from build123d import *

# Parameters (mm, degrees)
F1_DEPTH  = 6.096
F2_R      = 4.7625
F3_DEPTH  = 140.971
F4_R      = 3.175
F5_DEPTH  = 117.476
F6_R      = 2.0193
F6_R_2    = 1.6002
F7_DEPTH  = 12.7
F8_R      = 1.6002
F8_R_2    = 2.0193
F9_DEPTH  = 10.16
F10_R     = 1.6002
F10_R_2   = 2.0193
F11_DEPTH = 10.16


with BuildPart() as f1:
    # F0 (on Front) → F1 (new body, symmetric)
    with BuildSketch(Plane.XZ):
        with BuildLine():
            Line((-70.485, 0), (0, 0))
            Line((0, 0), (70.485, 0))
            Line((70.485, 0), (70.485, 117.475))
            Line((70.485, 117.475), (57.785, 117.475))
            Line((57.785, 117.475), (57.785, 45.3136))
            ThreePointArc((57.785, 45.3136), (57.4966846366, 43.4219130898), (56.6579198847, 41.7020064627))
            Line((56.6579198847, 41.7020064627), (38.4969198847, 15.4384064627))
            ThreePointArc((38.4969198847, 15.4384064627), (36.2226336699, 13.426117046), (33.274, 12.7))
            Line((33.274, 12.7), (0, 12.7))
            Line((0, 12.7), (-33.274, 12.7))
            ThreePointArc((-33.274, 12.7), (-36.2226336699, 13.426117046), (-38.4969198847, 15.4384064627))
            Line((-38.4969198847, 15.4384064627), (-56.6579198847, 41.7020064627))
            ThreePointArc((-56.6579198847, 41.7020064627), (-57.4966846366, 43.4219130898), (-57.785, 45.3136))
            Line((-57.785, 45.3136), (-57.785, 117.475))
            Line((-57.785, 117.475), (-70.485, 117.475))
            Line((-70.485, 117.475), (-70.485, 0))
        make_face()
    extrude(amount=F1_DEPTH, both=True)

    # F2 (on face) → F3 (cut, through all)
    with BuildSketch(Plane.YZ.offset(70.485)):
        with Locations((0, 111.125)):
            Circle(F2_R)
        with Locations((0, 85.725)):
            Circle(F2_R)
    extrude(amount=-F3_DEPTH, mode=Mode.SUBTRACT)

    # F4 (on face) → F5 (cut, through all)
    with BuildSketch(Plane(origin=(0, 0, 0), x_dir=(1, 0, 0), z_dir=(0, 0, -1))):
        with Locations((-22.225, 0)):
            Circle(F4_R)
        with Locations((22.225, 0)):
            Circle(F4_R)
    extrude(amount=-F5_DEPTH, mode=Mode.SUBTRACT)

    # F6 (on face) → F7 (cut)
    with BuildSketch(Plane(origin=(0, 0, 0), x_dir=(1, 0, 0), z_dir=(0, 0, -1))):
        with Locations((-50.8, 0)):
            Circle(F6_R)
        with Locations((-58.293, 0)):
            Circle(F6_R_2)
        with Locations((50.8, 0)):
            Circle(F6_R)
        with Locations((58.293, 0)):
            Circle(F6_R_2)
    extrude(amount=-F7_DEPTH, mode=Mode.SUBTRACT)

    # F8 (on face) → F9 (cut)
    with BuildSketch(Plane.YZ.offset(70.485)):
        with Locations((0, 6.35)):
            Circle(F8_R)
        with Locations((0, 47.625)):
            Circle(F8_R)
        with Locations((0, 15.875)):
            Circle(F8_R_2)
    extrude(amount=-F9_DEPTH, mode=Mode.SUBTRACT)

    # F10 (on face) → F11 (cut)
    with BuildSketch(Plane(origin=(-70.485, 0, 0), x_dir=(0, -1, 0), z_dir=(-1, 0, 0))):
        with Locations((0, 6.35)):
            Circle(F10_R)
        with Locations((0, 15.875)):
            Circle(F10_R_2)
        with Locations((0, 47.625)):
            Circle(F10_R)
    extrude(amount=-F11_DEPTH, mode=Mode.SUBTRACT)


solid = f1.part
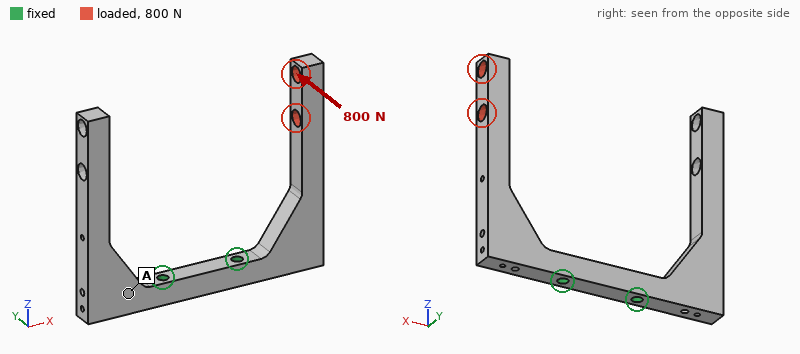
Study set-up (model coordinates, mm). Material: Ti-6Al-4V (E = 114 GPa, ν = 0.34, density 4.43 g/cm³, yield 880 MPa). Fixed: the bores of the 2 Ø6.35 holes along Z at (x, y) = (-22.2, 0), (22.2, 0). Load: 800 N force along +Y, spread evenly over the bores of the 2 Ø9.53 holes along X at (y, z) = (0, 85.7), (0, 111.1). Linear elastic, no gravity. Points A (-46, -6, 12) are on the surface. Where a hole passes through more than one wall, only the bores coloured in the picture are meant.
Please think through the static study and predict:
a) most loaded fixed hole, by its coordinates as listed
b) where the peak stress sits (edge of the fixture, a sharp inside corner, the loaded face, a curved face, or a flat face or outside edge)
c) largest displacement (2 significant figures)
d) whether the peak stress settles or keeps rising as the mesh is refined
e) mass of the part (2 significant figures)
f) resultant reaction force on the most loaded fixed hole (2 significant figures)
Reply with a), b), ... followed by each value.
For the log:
a) (22.2, 0)
b) edge of the fixture
c) 2.1 mm
d) keeps rising
e) 250 g
f) 890 N
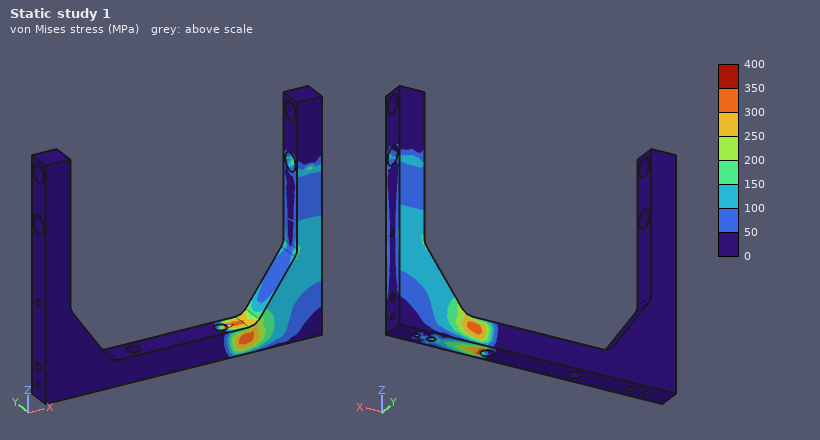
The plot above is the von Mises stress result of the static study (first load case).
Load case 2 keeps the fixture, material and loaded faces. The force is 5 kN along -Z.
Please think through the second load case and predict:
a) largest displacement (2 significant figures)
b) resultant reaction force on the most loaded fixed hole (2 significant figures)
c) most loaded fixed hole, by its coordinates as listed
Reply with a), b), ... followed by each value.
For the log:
a) 1.6 mm
b) 5.1 kN
c) (22.2, 0)
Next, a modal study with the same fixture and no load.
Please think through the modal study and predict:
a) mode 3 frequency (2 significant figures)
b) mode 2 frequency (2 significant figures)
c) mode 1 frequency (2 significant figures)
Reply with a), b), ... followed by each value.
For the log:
a) 860 Hz
b) 670 Hz
c) 670 Hz
